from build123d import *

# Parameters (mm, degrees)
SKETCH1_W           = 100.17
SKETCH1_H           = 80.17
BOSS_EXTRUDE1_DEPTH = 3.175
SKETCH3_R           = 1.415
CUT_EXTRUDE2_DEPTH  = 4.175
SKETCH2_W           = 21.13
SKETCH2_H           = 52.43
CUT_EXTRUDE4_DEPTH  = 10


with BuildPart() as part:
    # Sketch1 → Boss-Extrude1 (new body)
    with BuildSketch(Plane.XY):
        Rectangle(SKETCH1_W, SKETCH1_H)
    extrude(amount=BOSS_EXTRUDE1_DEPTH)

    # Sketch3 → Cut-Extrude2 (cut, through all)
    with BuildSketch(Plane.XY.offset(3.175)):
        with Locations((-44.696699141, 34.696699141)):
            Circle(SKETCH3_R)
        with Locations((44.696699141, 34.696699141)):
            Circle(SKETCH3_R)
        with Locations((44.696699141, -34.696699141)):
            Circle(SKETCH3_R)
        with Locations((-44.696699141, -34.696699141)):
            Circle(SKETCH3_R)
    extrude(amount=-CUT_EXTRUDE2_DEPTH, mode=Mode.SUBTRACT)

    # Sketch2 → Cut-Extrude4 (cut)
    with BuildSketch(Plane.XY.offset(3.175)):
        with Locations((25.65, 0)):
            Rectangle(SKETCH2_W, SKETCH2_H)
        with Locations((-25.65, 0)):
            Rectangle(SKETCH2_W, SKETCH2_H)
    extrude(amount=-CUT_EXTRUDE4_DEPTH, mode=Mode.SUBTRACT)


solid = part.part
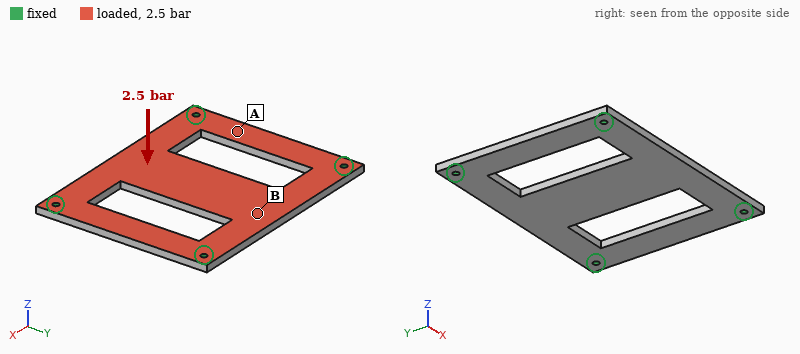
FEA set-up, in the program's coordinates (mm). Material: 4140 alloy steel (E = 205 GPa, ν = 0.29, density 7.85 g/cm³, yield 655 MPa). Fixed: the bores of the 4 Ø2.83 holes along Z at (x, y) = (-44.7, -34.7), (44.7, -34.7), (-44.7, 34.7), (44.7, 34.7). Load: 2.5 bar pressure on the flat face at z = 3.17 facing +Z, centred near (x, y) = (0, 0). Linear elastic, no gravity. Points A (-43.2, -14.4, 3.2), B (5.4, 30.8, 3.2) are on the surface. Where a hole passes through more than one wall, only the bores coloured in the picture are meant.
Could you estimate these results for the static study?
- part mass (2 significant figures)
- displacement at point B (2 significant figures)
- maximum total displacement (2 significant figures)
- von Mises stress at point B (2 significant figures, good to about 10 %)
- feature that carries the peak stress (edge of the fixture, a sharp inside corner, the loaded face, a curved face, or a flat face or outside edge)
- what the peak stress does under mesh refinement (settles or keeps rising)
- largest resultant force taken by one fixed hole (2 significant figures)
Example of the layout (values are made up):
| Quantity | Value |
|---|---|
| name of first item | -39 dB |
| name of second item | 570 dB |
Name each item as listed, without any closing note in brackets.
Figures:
| Quantity | Value |
|---|---|
| part mass | 140 g |
| displacement at point B | 0.13 mm |
| maximum total displacement | 0.18 mm |
| von Mises stress at point B | 62 MPa |
| feature that carries the peak stress | edge of the fixture |
| what the peak stress does under mesh refinement | keeps rising |
| largest resultant force taken by one fixed hole | 360 N |
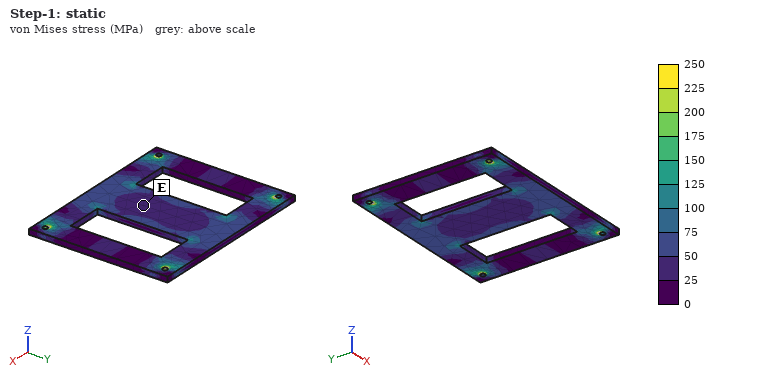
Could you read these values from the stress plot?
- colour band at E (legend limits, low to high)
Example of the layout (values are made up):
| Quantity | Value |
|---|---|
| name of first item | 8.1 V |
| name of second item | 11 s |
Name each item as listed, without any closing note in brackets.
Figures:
| Quantity | Value |
|---|---|
| colour band at E | 25 to 50 MPa |
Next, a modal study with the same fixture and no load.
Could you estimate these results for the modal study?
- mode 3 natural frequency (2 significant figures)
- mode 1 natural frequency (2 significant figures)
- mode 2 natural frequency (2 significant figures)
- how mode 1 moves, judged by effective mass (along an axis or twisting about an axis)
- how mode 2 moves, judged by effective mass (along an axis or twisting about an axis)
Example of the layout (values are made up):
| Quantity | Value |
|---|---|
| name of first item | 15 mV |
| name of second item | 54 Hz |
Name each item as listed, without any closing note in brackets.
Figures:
| Quantity | Value |
|---|---|
| mode 3 natural frequency | 3400 Hz |
| mode 1 natural frequency | 1400 Hz |
| mode 2 natural frequency | 2200 Hz |
| how mode 1 moves, judged by effective mass | along Z |
| how mode 2 moves, judged by effective mass | twisting about X |
